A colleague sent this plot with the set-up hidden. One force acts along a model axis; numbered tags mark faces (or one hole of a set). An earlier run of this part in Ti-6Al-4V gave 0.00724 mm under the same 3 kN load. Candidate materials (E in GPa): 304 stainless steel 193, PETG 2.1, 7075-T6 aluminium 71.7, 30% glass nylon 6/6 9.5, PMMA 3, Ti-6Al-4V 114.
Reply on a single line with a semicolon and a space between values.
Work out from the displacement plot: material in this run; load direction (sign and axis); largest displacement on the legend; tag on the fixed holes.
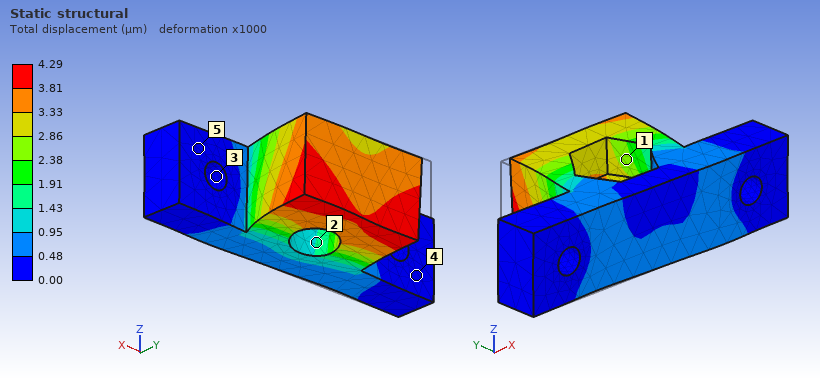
304 stainless steel; +X; 4.29 µm; 3
